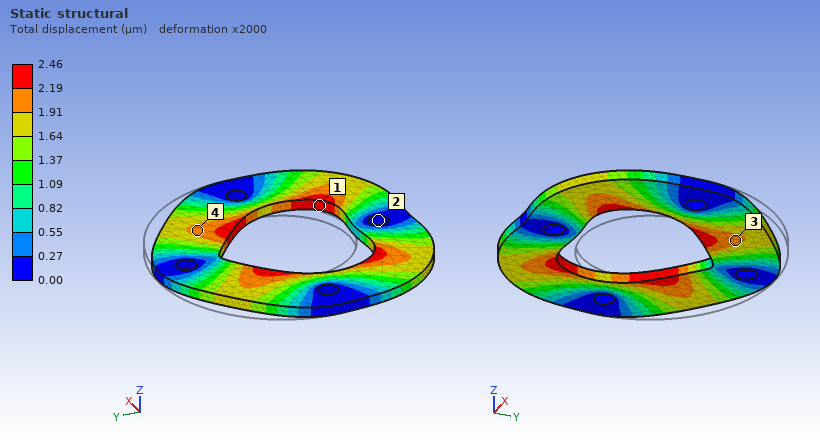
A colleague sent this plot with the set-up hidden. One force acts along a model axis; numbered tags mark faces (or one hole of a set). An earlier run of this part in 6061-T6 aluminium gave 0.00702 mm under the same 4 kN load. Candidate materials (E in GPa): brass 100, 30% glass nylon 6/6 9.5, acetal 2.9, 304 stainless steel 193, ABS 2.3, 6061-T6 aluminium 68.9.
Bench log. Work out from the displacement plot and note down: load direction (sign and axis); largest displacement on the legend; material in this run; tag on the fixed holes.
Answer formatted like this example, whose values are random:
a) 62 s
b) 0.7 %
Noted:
a) -Y
b) 2.46 µm
c) 304 stainless steel
d) 2
